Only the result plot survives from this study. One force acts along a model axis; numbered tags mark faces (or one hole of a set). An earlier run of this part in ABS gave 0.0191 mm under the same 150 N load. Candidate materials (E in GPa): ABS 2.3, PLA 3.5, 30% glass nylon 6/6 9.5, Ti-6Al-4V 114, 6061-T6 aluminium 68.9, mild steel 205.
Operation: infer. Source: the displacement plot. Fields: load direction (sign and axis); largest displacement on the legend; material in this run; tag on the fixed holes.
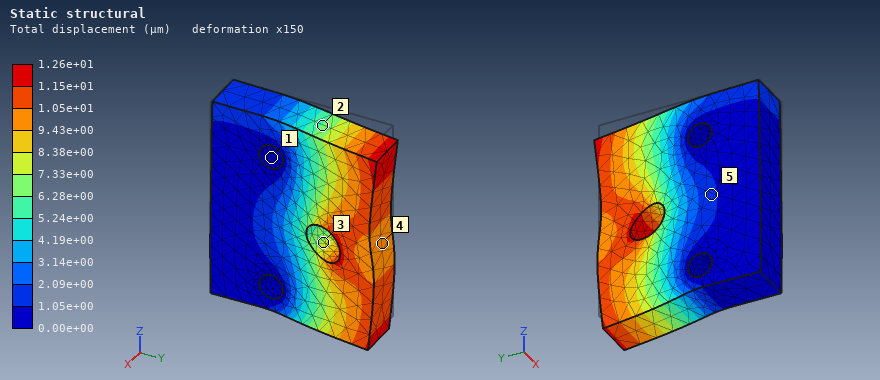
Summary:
-Z
1.26e+01 µm
PLA
1
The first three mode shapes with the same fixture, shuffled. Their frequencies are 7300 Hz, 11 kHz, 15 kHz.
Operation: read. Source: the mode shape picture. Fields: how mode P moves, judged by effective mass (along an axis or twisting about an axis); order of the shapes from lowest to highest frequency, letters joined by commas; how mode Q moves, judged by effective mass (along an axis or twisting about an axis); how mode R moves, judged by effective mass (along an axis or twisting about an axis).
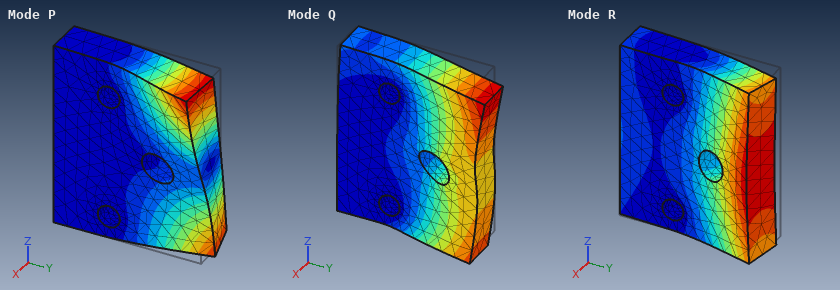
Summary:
twisting about Y
R, P, Q
along Z
along X
